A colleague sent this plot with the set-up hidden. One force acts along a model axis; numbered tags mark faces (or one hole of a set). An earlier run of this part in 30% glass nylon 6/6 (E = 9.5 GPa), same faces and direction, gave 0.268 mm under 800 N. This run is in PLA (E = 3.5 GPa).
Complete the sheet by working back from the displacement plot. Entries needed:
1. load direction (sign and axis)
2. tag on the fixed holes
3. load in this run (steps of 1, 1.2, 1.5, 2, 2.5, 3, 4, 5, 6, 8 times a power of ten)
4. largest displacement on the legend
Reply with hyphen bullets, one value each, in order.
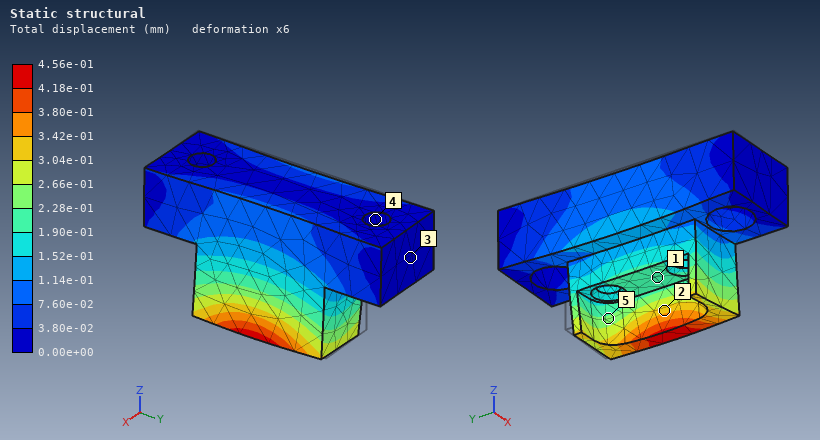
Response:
- +X
- 4
- 500 N
- 4.56e-01 mm
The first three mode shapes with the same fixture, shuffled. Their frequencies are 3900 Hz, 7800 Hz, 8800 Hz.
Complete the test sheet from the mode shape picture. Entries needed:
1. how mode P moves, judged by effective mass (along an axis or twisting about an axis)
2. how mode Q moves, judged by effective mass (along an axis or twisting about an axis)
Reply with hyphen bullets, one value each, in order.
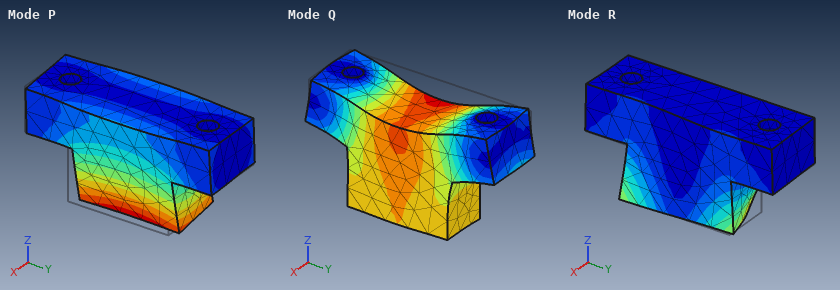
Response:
- along X
- along Z
